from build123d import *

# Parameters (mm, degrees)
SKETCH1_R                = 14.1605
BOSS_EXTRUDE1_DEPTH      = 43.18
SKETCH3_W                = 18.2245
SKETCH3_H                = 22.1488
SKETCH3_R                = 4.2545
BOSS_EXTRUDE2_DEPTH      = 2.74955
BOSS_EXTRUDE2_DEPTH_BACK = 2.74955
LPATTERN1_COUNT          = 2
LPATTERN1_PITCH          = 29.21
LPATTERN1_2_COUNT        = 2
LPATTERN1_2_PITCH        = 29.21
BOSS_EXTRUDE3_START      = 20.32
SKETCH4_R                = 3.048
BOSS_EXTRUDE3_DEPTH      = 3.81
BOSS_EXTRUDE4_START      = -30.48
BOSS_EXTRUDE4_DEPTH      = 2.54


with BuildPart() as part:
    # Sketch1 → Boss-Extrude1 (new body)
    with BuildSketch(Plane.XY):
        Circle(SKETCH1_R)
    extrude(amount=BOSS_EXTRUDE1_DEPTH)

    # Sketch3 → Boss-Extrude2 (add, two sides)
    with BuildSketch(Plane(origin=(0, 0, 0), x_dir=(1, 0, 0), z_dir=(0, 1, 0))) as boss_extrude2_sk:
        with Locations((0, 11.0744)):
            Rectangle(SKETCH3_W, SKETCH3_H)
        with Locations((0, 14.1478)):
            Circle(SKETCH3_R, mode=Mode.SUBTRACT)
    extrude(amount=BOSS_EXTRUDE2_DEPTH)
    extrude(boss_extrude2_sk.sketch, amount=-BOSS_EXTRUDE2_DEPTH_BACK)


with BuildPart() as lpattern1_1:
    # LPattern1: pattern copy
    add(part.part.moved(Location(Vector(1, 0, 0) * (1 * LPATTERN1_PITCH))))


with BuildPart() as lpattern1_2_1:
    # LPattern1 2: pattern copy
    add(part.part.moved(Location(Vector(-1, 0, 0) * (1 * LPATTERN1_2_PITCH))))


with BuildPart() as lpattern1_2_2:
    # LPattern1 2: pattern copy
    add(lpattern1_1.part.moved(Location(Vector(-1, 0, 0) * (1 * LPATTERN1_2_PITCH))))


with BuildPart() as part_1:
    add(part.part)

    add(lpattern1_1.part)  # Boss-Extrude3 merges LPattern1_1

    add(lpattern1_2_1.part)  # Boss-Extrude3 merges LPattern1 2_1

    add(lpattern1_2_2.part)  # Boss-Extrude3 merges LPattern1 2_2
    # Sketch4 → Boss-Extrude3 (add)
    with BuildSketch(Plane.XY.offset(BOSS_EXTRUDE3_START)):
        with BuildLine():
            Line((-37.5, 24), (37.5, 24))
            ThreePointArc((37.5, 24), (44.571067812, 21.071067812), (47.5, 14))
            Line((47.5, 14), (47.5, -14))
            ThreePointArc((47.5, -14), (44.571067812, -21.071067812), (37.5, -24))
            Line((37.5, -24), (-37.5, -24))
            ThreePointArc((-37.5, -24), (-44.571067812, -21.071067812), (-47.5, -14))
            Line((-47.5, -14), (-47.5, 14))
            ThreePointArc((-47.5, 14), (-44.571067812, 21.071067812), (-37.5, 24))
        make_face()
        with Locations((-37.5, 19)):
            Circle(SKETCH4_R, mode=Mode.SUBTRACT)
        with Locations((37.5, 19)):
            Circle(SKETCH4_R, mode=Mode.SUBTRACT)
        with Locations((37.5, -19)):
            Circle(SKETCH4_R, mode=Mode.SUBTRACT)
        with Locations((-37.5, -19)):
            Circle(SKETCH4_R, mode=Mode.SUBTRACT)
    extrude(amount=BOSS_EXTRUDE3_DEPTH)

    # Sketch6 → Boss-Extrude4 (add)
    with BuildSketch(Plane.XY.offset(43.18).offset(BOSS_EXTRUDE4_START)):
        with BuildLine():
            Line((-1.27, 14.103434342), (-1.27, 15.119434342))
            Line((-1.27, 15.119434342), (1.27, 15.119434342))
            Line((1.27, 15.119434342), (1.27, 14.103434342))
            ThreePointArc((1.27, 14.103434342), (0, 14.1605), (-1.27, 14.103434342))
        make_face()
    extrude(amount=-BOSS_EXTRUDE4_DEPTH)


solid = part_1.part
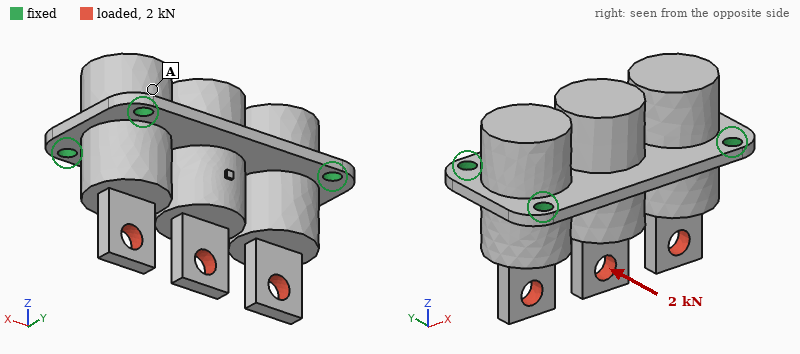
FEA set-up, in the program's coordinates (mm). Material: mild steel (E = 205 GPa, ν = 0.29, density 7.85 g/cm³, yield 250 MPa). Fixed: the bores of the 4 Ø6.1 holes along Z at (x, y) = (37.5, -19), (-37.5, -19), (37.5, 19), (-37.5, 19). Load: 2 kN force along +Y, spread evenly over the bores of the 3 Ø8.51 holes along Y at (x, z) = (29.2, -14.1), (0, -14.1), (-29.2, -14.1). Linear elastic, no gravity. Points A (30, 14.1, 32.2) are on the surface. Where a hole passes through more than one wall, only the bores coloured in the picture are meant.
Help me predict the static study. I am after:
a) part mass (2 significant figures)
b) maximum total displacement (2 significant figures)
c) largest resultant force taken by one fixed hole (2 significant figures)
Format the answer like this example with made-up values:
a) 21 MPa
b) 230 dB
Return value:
a) 760 g
b) 64 µm
c) 1.3 kN
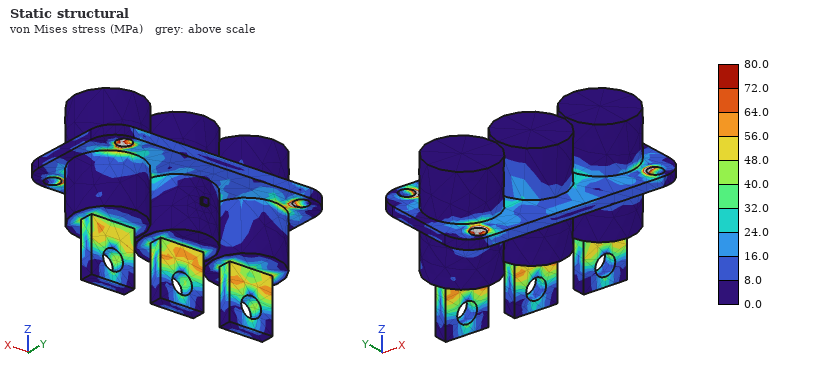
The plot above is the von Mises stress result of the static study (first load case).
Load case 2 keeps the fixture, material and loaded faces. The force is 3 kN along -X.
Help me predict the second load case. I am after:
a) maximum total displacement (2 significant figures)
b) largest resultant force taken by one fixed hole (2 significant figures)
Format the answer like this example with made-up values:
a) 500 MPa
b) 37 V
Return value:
a) 26 µm
b) 1.1 kN
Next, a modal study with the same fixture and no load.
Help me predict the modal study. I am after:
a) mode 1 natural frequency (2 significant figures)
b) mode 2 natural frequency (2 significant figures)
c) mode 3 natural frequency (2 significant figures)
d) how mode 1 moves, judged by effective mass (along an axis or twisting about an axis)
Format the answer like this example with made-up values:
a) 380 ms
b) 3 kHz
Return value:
a) 1900 Hz
b) 3000 Hz
c) 4000 Hz
d) along Z
